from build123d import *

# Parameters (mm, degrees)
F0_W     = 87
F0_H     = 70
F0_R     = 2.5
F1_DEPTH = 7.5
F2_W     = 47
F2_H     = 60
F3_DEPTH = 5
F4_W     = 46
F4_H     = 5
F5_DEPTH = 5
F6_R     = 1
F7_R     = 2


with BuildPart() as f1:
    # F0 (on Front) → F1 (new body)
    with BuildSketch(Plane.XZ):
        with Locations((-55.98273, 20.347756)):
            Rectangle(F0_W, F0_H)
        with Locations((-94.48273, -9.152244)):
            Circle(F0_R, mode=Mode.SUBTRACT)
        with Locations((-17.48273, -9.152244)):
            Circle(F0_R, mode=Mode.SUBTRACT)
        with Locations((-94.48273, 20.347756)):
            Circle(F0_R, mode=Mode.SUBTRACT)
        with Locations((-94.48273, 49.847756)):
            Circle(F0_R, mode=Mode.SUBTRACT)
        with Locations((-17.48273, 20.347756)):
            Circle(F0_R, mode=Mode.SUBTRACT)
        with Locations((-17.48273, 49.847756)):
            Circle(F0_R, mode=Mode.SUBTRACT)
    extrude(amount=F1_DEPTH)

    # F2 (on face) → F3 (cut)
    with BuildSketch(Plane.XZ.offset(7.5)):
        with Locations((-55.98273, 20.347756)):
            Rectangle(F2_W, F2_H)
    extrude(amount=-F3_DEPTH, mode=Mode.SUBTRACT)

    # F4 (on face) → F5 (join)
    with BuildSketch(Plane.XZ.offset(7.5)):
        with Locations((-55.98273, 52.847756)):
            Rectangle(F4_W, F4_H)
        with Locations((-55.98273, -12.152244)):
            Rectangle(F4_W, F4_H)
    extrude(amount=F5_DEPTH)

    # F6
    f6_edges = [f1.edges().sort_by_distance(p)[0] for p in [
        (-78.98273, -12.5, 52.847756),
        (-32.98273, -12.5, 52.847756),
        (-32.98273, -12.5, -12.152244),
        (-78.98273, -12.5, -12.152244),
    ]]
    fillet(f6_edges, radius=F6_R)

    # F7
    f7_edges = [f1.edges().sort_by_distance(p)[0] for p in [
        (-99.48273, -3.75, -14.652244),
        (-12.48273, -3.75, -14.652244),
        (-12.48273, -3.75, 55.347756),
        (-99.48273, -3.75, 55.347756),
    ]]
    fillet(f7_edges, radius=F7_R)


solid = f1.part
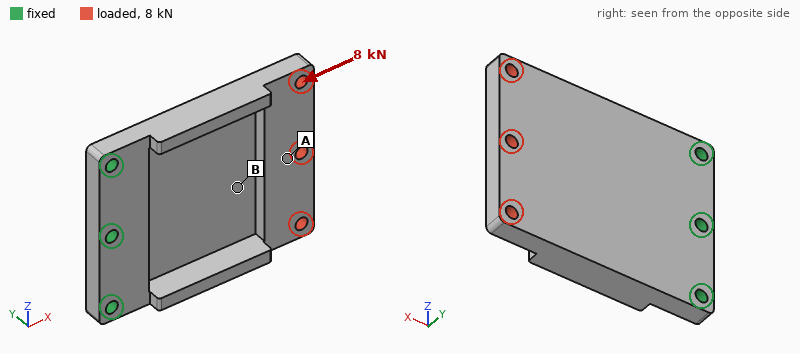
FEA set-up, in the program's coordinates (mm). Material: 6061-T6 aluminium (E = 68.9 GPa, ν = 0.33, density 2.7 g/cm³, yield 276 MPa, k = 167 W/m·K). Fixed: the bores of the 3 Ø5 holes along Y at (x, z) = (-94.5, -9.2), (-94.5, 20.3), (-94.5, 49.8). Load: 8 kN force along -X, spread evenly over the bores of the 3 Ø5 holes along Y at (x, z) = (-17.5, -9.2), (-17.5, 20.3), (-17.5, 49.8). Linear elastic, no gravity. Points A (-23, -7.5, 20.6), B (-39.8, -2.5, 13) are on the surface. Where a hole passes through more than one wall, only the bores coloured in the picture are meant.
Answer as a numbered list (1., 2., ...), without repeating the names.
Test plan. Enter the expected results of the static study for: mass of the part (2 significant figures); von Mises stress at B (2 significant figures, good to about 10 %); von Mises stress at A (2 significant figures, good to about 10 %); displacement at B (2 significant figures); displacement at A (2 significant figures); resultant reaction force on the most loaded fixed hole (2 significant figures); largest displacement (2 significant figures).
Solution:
1. 89 g
2. 49 MPa
3. 18 MPa
4. 0.092 mm
5. 0.20 mm
6. 3.1 kN
7. 0.27 mm
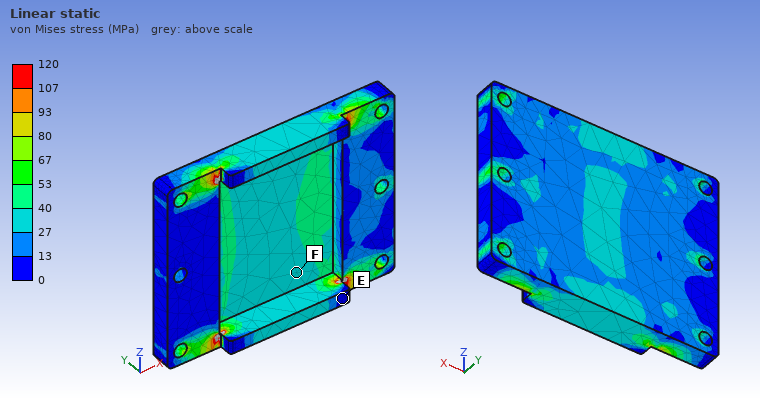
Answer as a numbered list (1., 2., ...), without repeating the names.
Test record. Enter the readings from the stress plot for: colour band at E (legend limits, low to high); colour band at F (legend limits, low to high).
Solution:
1. 0 to 13 MPa
2. 27 to 40 MPa
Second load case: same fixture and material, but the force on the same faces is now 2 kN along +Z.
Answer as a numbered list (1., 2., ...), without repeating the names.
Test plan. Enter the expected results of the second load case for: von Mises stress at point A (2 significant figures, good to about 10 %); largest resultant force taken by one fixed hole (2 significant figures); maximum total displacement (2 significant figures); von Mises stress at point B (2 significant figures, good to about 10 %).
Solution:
1. 26 MPa
2. 2.6 kN
3. 0.18 mm
4. 36 MPa
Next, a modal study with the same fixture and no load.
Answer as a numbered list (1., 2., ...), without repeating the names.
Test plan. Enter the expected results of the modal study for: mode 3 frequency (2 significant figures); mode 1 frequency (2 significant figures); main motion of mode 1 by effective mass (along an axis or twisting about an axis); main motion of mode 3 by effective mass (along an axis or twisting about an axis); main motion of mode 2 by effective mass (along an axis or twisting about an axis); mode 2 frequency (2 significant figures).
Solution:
1. 5000 Hz
2. 760 Hz
3. along Y
4. along Z
5. twisting about X
6. 1600 Hz
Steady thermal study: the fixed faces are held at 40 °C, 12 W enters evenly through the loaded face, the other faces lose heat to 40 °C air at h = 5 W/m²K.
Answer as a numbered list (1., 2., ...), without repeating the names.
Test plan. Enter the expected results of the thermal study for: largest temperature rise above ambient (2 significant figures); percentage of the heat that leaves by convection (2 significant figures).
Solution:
1. 19 K
2. 6.0 %
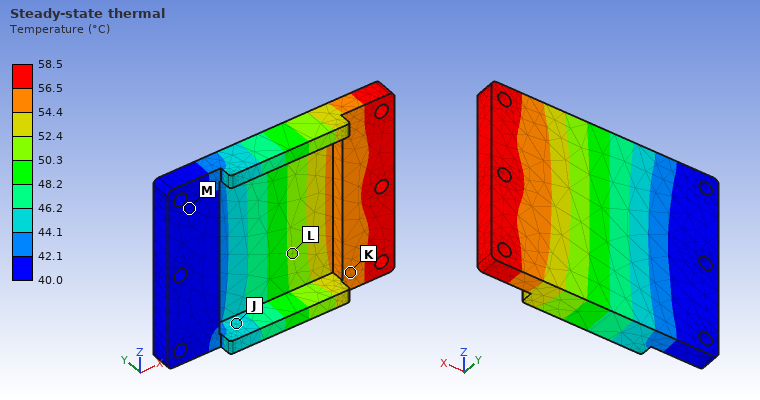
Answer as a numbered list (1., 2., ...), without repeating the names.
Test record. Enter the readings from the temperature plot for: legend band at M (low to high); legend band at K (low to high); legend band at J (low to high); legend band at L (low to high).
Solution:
1. 40.0 to 42.1 °C
2. 54.4 to 56.5 °C
3. 44.1 to 46.2 °C
4. 50.3 to 52.4 °C
